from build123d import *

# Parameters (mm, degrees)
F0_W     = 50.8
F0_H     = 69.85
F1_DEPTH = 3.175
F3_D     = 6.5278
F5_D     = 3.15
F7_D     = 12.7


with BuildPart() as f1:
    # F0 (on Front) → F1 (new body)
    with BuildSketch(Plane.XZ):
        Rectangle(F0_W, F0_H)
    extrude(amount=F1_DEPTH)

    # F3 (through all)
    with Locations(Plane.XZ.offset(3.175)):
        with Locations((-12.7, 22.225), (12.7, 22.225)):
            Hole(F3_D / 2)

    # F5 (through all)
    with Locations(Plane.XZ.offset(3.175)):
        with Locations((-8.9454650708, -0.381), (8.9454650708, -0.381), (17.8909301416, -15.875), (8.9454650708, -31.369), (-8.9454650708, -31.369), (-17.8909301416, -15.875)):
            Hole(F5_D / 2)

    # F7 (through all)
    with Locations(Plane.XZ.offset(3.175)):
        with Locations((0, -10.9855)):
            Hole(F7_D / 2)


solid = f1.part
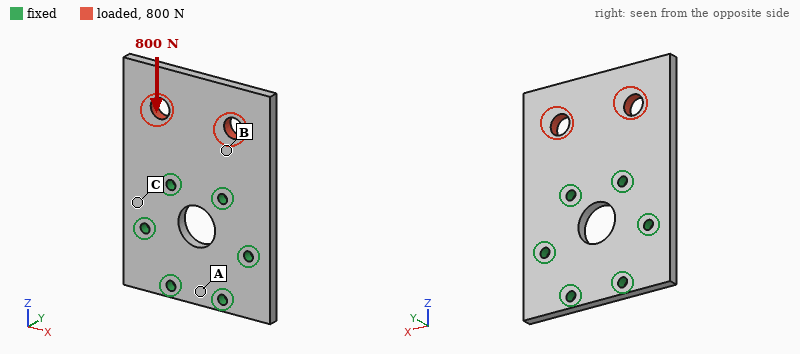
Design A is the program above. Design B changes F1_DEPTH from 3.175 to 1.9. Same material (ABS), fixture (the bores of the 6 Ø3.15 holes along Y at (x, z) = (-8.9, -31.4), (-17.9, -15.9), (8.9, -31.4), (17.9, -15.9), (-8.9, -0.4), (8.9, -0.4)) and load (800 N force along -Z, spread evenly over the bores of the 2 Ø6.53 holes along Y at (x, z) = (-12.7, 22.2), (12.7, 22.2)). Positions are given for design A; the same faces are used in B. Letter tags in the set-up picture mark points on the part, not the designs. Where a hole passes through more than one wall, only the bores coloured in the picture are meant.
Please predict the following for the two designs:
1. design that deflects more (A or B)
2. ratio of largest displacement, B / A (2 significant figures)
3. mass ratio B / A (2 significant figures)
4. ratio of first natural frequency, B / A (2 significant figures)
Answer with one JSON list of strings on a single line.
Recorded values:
["B", "1.7", "0.60", "0.61"]
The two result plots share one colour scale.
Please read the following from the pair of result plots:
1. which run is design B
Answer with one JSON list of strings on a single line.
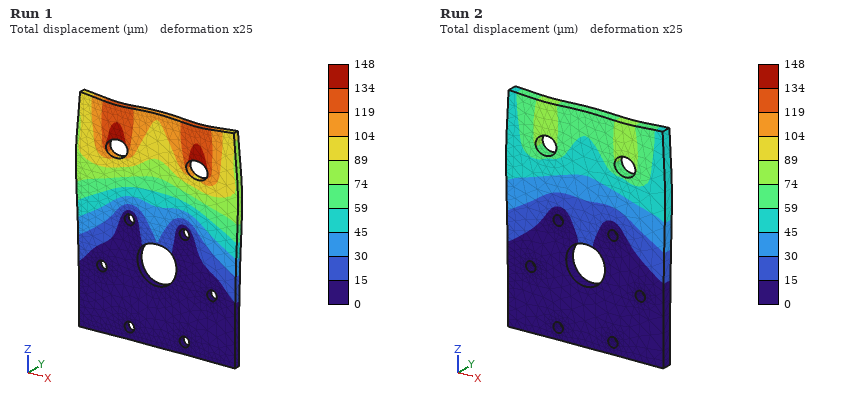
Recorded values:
["Run 1"]
